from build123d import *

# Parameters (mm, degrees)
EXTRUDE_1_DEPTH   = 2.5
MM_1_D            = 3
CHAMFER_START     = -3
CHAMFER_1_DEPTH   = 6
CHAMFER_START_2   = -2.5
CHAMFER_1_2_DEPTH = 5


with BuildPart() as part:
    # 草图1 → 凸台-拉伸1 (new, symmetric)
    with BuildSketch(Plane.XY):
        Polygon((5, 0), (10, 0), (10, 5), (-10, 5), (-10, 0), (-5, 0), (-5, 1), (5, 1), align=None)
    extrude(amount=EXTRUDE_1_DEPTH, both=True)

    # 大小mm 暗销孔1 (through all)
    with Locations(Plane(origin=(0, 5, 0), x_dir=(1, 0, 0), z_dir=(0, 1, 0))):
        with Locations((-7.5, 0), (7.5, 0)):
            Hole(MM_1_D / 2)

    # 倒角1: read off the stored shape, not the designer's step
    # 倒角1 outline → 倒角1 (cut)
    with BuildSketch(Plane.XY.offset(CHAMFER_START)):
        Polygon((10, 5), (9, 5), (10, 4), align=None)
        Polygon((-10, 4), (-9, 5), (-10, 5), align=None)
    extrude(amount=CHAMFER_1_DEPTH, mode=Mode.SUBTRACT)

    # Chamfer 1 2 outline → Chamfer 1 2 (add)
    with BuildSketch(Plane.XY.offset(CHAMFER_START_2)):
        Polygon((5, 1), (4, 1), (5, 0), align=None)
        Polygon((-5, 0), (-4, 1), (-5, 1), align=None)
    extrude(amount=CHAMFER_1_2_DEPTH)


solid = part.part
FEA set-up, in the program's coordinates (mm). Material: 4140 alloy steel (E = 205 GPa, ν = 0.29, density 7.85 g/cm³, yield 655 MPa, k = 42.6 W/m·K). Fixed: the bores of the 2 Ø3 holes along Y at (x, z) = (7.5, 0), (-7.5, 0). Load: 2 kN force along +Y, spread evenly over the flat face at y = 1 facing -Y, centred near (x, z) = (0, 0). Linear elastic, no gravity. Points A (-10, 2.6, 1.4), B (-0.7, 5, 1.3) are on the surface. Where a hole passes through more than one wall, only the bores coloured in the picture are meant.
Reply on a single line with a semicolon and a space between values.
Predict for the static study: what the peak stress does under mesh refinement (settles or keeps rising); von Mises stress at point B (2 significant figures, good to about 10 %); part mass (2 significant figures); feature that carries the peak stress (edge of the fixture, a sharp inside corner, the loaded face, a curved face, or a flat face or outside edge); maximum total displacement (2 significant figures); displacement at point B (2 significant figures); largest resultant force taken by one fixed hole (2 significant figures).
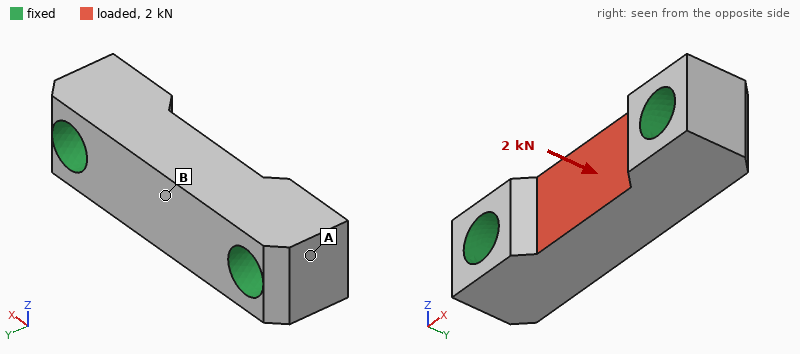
keeps rising; 110 MPa; 3.0 g; edge of the fixture; 5.4 µm; 4.5 µm; 1.0 kN
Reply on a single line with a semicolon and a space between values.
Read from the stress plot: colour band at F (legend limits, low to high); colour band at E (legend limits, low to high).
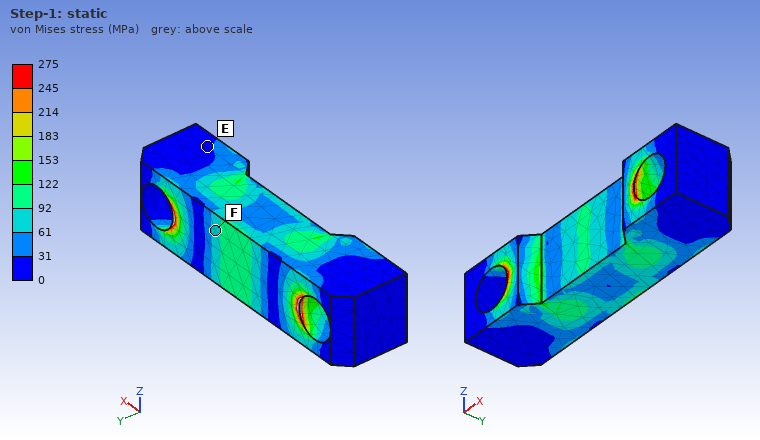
61 to 92 MPa; 0 to 31 MPa
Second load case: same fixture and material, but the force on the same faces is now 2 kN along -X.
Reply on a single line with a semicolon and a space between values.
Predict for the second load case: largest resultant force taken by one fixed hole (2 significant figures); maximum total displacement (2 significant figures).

1.0 kN; 2.1 µm
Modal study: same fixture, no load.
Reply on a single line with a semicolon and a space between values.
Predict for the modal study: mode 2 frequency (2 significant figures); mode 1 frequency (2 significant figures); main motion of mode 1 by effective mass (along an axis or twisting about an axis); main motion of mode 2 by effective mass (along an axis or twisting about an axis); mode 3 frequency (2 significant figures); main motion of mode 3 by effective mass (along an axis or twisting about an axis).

95 kHz; 89 kHz; along Z; along Y; 120 kHz; twisting about X
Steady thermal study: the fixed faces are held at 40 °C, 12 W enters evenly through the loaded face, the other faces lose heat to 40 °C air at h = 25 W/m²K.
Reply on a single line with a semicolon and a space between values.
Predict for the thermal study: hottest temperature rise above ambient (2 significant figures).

38 K
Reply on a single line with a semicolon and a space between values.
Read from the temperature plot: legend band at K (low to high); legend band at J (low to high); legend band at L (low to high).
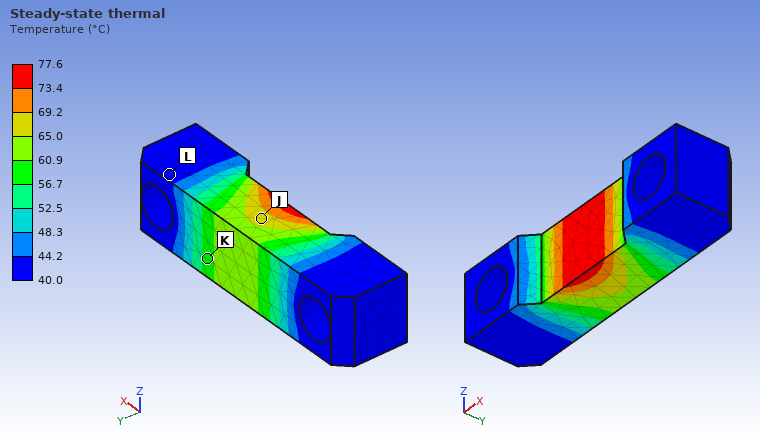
56.7 to 60.9 °C; 65.0 to 69.2 °C; 40.0 to 44.2 °C
